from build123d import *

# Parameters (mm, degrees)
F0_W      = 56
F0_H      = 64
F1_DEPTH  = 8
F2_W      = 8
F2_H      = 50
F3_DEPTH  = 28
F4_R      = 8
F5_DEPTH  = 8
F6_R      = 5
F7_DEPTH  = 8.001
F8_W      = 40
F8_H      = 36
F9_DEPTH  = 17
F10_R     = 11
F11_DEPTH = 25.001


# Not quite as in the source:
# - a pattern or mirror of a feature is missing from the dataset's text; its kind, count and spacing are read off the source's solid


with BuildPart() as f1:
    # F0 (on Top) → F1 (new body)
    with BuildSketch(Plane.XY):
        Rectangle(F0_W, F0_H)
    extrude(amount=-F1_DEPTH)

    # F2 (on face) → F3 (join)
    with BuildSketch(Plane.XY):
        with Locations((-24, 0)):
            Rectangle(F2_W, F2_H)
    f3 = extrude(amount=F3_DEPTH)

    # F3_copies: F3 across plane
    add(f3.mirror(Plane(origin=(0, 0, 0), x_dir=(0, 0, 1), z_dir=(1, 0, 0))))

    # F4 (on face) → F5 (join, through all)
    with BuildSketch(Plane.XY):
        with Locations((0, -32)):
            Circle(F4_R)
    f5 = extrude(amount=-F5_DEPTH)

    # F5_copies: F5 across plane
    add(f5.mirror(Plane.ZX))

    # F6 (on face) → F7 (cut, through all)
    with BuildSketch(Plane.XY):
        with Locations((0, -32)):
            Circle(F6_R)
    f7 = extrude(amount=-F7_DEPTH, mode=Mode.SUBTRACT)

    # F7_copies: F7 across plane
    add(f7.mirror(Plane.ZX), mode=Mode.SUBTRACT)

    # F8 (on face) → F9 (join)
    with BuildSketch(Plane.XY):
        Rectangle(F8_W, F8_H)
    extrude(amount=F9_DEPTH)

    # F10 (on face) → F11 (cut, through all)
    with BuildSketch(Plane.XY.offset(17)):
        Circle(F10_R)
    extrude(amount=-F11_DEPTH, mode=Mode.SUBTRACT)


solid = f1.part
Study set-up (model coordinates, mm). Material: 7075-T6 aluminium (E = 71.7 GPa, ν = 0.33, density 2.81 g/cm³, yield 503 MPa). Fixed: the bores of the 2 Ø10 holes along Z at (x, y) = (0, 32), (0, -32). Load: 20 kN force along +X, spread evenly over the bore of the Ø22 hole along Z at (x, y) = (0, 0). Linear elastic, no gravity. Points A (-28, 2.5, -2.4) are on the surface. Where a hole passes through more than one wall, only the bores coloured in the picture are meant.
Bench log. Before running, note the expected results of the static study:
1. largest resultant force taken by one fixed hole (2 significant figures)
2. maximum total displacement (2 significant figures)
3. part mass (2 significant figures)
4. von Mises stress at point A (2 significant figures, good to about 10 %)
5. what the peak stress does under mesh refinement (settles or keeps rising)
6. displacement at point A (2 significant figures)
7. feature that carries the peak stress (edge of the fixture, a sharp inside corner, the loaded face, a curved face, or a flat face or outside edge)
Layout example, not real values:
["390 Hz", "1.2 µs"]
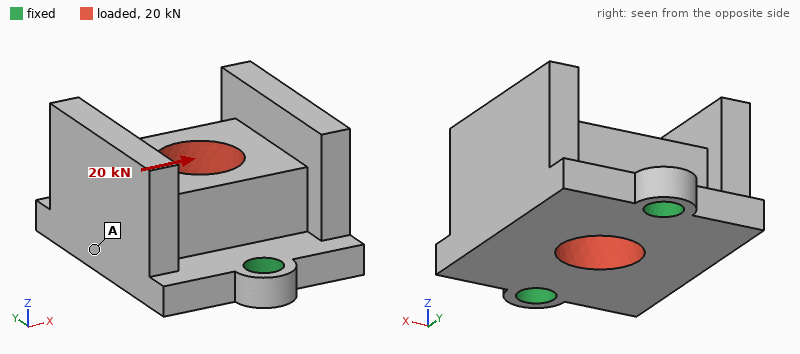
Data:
["10 kN", "0.27 mm", "190 g", "40 MPa", "keeps rising", "0.16 mm", "edge of the fixture"]
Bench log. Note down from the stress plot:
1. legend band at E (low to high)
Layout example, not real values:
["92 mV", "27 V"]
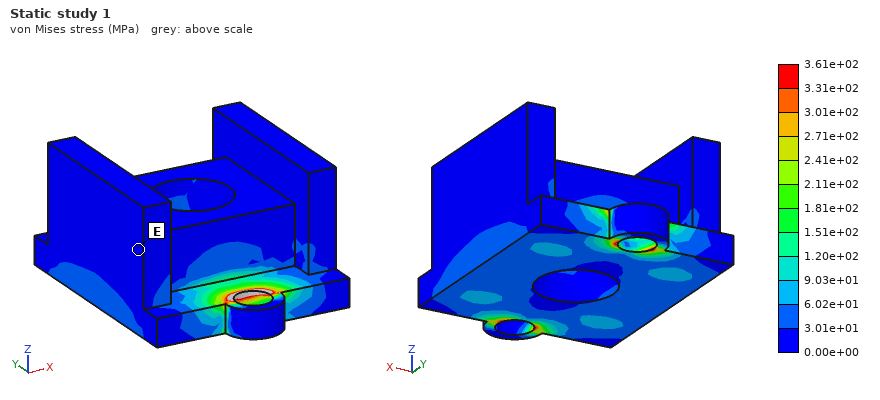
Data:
["0.00e+00 to 3.01e+01 MPa"]
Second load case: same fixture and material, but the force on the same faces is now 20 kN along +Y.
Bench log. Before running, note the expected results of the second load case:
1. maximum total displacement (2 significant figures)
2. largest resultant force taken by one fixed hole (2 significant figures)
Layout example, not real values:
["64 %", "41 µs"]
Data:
["40 µm", "11 kN"]
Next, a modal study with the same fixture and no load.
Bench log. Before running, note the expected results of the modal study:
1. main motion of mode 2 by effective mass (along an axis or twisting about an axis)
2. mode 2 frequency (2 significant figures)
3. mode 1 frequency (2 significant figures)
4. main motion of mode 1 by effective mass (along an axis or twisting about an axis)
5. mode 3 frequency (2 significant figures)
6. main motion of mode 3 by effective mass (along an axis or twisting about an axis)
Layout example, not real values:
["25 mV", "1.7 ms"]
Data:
["along Z", "6500 Hz", "2800 Hz", "along X", "8200 Hz", "along Y"]
